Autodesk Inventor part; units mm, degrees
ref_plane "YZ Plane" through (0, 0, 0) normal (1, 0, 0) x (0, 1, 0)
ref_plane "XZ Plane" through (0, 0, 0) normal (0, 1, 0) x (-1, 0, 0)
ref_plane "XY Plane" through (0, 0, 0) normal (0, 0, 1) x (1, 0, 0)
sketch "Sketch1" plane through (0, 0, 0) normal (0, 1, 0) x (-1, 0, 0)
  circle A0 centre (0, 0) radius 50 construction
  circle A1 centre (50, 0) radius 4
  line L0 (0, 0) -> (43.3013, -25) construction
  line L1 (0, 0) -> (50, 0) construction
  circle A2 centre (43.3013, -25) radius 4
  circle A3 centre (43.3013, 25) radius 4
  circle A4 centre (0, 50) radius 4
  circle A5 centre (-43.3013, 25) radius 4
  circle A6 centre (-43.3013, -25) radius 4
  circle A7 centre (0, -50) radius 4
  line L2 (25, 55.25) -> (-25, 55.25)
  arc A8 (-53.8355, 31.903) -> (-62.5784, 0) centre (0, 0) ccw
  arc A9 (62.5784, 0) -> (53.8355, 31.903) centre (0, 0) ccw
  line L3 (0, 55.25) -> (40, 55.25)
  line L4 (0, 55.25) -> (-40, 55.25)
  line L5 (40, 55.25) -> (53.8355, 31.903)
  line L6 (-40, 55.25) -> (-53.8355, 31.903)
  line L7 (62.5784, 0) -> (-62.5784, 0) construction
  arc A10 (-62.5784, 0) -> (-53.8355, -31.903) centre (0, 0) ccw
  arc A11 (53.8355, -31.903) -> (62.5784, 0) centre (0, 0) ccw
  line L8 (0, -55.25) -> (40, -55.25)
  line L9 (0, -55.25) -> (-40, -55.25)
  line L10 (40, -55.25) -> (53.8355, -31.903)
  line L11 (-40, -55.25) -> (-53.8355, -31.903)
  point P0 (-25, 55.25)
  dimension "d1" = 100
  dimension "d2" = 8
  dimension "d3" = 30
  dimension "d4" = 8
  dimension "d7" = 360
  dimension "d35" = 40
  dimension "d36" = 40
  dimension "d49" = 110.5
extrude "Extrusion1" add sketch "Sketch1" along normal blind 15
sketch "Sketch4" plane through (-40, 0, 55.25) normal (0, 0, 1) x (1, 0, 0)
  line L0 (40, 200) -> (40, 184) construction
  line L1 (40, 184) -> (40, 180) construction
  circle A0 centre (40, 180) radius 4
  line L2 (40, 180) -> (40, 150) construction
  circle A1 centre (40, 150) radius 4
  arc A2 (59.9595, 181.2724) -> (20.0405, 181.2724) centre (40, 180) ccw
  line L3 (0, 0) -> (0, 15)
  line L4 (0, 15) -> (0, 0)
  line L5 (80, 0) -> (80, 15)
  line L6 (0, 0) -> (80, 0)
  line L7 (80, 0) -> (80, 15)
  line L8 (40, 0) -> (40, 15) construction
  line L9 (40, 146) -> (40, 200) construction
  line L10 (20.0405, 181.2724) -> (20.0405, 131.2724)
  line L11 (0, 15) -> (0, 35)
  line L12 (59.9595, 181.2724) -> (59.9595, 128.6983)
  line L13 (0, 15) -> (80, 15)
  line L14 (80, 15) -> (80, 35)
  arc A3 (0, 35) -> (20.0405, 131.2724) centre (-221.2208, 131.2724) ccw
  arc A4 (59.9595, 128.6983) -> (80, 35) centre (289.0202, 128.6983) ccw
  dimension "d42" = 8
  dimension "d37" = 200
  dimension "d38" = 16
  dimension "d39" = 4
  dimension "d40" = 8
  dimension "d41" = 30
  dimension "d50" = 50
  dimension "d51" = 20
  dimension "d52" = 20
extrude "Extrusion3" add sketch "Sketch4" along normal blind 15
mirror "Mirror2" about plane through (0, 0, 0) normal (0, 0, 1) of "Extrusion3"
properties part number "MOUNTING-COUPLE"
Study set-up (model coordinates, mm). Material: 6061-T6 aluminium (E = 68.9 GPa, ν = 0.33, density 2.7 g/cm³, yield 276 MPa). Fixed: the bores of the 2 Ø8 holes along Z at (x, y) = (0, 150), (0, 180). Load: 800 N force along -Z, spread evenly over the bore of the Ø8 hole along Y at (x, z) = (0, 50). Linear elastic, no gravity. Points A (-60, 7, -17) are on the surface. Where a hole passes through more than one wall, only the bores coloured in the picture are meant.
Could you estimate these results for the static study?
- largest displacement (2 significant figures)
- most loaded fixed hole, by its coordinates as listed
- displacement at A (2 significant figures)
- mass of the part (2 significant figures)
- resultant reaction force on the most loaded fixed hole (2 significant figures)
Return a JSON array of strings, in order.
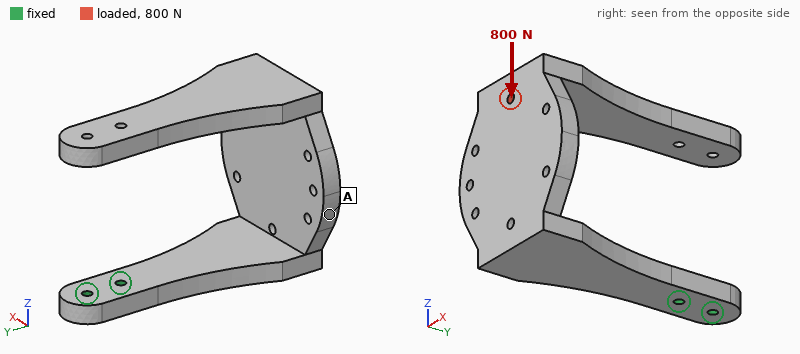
["1.6 mm", "(0, 150)", "1.0 mm", "1.3 kg", "2.0 kN"]
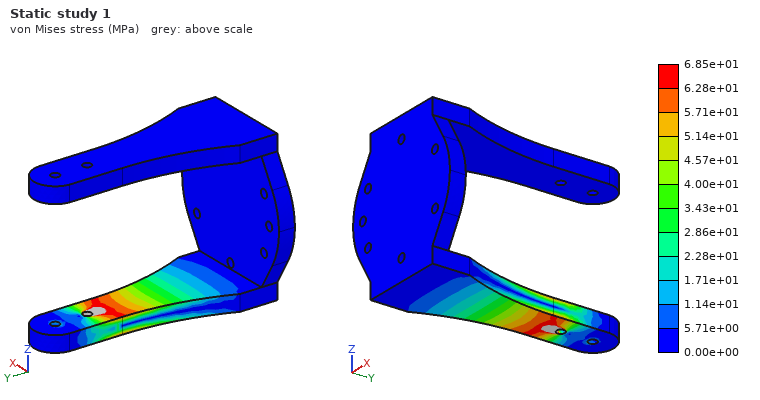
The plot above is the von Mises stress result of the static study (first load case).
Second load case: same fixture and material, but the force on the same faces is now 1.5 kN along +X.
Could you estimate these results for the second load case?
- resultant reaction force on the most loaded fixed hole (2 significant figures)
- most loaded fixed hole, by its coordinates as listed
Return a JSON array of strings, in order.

["6.4 kN", "(0, 150)"]
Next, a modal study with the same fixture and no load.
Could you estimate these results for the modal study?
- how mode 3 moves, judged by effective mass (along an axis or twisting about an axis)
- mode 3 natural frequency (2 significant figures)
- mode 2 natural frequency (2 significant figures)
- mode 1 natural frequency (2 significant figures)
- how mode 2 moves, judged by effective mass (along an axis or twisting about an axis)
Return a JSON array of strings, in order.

["along Z", "230 Hz", "140 Hz", "110 Hz", "along X"]
